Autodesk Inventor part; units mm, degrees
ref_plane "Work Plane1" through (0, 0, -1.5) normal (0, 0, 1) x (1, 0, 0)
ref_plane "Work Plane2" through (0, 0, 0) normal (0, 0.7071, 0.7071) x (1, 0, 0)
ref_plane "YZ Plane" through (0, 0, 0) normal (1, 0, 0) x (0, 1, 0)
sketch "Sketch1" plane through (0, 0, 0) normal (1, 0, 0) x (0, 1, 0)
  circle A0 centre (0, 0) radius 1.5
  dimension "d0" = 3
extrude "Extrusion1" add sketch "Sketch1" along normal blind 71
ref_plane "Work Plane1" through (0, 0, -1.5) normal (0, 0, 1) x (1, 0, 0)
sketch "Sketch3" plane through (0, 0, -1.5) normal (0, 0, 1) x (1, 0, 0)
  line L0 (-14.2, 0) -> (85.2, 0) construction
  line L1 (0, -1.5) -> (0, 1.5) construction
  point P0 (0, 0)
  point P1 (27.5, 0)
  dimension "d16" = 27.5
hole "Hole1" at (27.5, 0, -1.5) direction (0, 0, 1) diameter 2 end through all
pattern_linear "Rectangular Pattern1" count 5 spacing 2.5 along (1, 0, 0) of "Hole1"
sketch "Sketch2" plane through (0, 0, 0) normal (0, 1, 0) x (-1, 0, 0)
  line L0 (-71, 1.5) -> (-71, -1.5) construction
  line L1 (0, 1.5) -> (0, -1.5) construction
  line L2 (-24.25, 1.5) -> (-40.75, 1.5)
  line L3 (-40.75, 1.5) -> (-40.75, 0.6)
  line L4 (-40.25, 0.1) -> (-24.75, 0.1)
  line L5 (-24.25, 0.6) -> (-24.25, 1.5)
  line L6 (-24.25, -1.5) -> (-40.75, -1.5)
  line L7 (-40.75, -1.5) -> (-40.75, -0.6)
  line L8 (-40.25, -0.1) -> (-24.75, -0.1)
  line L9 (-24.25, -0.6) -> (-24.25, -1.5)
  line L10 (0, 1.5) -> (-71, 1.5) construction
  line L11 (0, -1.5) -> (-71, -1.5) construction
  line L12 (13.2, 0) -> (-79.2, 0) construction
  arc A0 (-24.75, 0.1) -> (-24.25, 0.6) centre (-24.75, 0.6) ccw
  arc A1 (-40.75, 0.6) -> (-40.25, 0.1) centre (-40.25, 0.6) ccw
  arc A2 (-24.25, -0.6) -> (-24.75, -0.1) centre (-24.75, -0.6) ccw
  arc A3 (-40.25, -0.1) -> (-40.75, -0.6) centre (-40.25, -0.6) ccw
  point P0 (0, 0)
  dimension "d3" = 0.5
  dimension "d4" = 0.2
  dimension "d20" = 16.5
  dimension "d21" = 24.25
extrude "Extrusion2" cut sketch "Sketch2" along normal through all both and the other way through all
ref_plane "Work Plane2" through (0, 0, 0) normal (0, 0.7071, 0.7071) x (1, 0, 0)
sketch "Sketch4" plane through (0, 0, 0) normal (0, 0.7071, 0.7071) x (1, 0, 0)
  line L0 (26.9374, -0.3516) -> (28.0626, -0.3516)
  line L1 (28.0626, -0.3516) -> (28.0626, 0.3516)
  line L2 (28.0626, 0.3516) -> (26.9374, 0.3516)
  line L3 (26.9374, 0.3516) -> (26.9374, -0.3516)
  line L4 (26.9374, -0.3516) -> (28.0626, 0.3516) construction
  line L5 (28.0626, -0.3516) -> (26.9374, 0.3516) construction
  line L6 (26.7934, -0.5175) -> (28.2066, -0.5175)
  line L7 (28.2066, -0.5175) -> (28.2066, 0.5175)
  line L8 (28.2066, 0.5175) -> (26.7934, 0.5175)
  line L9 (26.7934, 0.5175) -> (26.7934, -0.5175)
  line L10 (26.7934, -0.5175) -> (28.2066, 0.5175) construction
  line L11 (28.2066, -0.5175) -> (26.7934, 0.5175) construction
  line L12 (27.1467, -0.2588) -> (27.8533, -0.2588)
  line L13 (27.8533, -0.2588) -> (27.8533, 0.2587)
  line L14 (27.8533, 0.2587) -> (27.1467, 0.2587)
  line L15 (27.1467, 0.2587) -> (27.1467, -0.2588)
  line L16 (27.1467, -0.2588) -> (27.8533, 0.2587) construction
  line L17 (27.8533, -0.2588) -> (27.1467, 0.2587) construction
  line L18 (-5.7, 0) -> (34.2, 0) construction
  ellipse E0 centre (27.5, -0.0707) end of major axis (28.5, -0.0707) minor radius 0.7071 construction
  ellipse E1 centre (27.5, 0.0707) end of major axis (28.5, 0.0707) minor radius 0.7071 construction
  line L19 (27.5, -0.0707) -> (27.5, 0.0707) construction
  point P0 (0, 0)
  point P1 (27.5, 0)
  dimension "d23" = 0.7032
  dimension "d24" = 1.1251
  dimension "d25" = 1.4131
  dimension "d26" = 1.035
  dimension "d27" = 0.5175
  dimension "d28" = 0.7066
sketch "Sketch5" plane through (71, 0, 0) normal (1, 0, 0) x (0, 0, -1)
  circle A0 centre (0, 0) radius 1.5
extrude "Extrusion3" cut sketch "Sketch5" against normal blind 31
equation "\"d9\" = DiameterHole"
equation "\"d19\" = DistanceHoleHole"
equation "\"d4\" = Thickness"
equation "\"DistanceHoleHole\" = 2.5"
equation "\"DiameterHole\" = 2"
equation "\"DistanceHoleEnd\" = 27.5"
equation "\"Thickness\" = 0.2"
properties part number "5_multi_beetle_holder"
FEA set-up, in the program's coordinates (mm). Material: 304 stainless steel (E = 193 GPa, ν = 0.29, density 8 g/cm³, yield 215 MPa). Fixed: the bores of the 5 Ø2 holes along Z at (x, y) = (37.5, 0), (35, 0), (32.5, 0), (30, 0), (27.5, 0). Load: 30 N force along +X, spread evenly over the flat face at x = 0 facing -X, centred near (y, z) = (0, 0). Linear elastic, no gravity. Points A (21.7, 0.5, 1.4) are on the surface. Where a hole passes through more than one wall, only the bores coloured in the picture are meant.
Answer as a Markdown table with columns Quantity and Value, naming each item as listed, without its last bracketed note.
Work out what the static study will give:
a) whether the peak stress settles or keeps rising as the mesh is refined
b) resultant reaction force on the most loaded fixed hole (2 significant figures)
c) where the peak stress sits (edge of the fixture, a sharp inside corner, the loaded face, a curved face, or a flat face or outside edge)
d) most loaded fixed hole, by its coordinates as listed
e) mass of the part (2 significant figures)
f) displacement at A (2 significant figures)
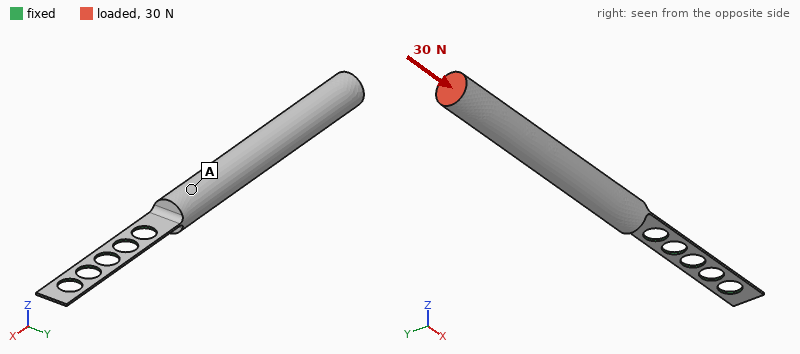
| Quantity | Value |
|---|---|
| whether the peak stress settles or keeps rising as the mesh is refined | keeps rising |
| resultant reaction force on the most loaded fixed hole | 30 N |
| where the peak stress sits | edge of the fixture |
| most loaded fixed hole, by its coordinates as listed | (27.5, 0) |
| mass of the part | 1.4 g |
| displacement at A | 0.72 µm |
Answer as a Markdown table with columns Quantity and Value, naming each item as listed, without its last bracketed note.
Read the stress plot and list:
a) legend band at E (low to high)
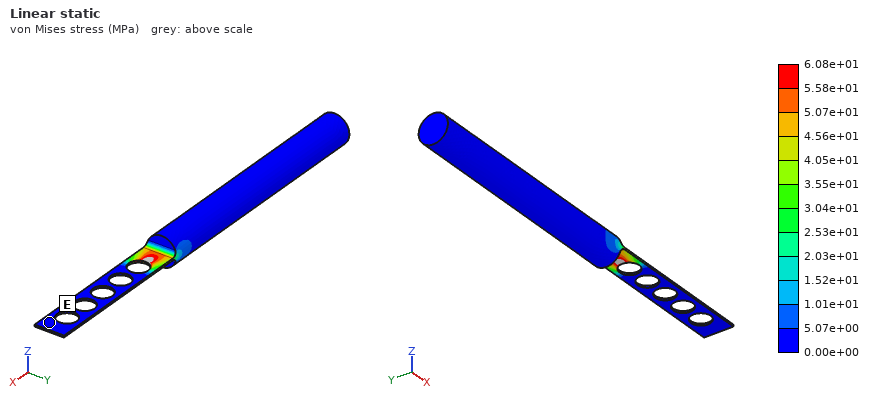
| Quantity | Value |
|---|---|
| legend band at E | 0.00e+00 to 5.07e+00 MPa |
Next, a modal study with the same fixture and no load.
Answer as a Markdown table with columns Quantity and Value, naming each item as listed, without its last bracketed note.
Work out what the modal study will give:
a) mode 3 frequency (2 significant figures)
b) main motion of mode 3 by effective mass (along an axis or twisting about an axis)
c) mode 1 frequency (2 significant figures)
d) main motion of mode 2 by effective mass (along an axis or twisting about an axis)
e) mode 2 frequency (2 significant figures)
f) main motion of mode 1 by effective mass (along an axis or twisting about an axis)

| Quantity | Value |
|---|---|
| mode 3 frequency | 2900 Hz |
| main motion of mode 3 by effective mass | twisting about X |
| mode 1 frequency | 130 Hz |
| main motion of mode 2 by effective mass | along Y |
| mode 2 frequency | 1400 Hz |
| main motion of mode 1 by effective mass | along Z |
